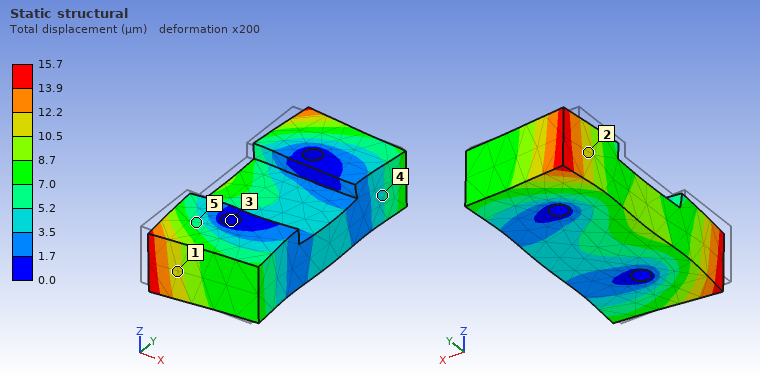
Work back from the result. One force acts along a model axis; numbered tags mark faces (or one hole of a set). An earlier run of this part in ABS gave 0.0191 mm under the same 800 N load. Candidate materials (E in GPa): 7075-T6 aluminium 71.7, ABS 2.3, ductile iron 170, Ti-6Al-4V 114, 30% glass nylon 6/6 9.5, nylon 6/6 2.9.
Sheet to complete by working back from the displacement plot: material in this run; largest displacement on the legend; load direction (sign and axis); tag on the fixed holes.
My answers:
nylon 6/6
15.7 µm
+X
3
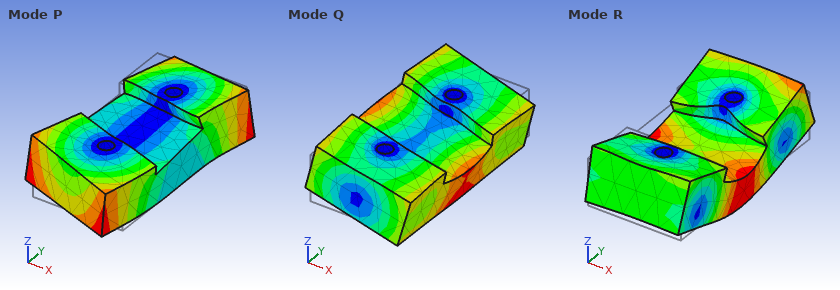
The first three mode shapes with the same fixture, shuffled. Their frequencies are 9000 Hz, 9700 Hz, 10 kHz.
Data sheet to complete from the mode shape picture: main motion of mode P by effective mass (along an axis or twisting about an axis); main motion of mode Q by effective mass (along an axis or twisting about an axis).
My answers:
twisting about Z
twisting about Y
